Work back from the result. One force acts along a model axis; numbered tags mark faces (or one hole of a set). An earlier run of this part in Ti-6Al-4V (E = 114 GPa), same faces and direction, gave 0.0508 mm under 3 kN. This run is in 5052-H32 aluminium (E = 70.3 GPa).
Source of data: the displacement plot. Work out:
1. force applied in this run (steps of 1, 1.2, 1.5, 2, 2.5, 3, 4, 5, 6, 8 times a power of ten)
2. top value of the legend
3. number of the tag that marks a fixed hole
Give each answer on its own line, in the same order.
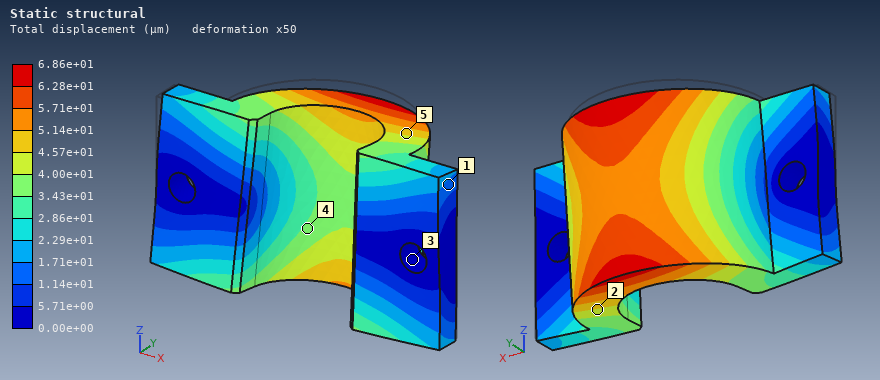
2.5 kN
6.86e+01 µm
3
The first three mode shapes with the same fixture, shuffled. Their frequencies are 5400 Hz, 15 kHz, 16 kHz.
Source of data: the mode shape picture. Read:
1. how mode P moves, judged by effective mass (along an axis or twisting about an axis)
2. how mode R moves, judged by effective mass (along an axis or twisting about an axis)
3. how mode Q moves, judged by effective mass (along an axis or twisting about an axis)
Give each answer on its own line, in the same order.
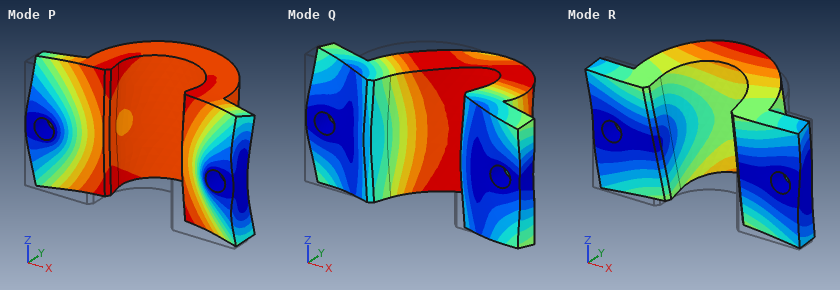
along Y
along Z
along X
